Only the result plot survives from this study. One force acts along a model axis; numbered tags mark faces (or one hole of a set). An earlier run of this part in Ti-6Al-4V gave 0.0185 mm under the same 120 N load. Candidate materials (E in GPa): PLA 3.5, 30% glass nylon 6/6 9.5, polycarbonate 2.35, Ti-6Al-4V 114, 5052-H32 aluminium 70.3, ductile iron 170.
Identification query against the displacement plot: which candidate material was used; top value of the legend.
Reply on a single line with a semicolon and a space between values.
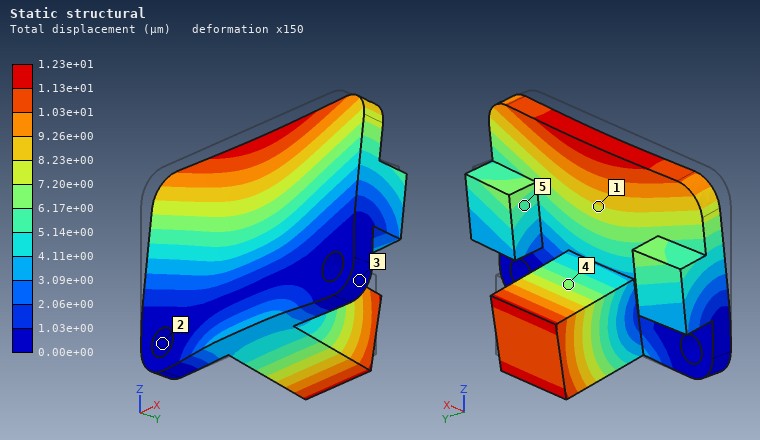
ductile iron; 1.23e+01 µm
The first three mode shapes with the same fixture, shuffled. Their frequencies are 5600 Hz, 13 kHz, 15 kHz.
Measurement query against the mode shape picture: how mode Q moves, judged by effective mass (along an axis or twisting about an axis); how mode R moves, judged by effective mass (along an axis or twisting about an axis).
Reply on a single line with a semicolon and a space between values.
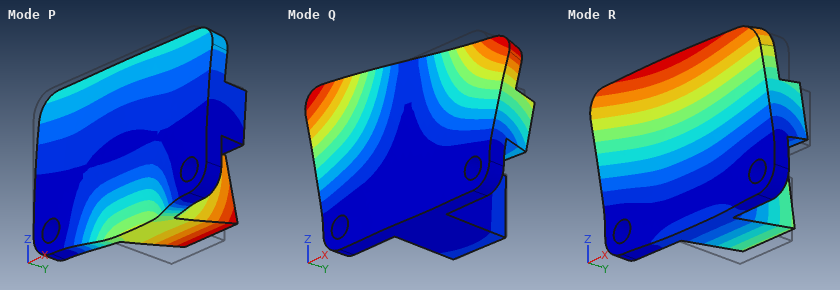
twisting about Z; along Y
